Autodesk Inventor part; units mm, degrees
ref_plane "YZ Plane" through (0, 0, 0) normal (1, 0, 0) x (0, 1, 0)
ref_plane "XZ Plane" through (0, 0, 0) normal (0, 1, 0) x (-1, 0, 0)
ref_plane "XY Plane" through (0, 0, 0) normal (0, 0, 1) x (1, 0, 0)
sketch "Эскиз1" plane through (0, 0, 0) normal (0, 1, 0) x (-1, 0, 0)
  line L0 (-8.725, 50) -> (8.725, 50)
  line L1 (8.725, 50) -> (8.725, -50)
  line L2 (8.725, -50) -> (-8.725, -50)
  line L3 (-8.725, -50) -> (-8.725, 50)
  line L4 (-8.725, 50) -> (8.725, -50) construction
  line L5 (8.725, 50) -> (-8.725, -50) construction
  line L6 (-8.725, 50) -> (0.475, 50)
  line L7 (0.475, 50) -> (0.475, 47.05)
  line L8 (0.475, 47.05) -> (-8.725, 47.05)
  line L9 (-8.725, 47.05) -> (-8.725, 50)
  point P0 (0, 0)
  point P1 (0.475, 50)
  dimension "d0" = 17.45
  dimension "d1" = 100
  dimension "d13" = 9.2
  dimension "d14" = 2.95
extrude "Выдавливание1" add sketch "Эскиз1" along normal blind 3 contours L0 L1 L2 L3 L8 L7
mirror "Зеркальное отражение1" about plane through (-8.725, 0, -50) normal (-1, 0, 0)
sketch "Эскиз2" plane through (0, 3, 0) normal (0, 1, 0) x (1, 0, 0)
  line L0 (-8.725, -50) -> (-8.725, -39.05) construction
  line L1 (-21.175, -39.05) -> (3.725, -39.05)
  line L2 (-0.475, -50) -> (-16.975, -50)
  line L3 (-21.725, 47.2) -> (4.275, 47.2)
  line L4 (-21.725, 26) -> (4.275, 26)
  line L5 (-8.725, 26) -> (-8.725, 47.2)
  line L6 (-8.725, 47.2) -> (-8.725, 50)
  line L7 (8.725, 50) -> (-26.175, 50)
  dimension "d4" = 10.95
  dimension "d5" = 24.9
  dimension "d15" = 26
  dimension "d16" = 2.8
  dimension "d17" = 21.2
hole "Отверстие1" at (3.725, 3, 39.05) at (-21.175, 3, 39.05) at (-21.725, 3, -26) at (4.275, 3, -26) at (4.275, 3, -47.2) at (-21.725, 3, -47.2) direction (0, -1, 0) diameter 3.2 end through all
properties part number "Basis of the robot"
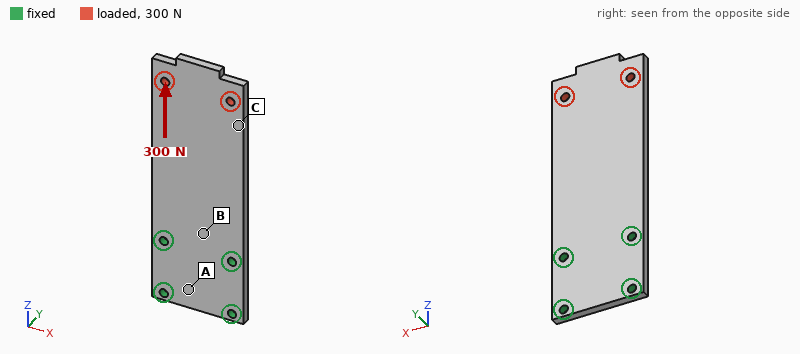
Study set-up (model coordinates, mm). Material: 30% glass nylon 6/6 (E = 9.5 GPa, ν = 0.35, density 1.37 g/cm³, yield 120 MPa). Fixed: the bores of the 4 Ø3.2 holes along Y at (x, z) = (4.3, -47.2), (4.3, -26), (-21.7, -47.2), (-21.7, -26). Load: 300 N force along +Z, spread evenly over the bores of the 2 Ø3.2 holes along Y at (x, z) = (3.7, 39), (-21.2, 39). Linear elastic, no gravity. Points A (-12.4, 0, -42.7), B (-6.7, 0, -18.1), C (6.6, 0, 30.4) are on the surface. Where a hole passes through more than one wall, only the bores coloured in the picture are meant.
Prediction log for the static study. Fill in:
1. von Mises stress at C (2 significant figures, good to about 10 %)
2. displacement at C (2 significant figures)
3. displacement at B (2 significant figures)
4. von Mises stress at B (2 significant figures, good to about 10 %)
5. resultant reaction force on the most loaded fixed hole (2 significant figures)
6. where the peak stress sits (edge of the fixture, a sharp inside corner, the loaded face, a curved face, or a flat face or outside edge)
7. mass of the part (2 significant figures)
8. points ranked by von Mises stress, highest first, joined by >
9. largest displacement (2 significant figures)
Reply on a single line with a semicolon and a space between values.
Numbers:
3.6 MPa; 19 µm; 4.1 µm; 2.0 MPa; 130 N; the loaded face; 14 g; C > B > A; 24 µm
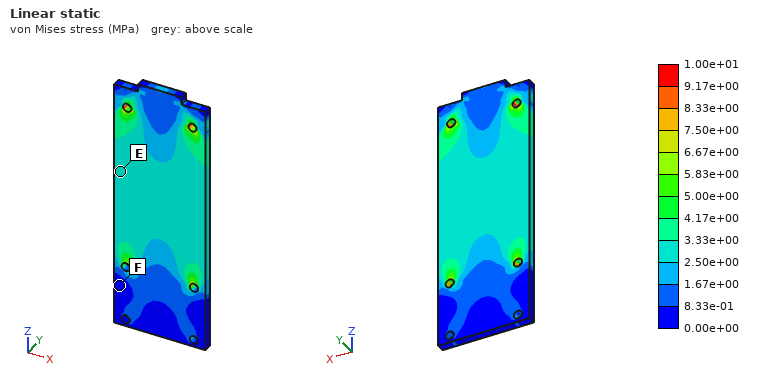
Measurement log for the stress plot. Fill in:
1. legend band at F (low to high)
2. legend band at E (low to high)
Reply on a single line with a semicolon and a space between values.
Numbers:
0.00e+00 to 8.33e-01 MPa; 2.50e+00 to 3.33e+00 MPa
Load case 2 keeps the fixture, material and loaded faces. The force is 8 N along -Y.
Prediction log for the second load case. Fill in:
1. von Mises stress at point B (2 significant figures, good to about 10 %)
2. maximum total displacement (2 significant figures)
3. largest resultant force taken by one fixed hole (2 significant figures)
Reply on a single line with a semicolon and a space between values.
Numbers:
7.5 MPa; 1.2 mm; 7.5 N
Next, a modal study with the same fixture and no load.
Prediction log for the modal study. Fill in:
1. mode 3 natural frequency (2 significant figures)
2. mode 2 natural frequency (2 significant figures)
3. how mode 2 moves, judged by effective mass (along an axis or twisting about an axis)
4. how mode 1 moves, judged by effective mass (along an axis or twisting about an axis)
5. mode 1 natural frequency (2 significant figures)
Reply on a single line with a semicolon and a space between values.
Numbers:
1400 Hz; 1100 Hz; twisting about Z; along Y; 230 Hz
